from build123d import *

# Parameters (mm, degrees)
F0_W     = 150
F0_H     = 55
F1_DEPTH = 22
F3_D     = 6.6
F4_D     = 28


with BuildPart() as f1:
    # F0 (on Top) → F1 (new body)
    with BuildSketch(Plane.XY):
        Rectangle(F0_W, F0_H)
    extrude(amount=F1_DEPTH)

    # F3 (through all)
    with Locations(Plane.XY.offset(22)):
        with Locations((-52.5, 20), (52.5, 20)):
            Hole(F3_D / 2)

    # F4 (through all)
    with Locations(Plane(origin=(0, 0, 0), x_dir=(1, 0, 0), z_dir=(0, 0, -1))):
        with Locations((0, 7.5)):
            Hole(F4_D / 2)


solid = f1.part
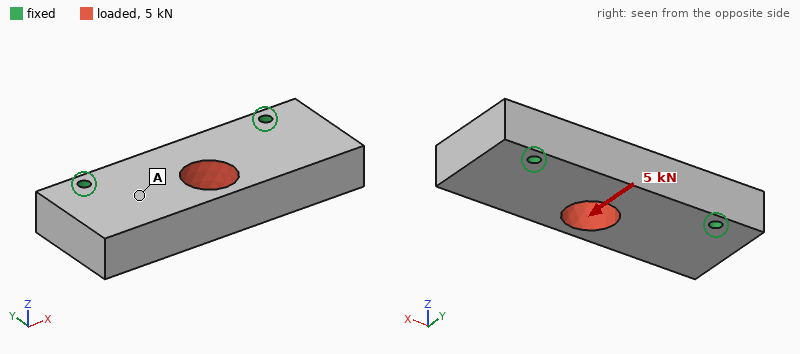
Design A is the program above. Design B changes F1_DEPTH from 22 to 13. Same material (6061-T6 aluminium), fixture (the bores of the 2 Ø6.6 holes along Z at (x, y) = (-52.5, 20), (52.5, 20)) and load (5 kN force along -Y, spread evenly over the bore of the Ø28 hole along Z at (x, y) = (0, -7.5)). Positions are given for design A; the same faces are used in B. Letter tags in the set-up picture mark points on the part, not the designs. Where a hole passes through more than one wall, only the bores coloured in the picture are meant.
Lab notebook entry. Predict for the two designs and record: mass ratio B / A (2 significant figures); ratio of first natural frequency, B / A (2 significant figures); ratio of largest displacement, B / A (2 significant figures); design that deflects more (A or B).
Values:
0.59
0.69
1.7
B
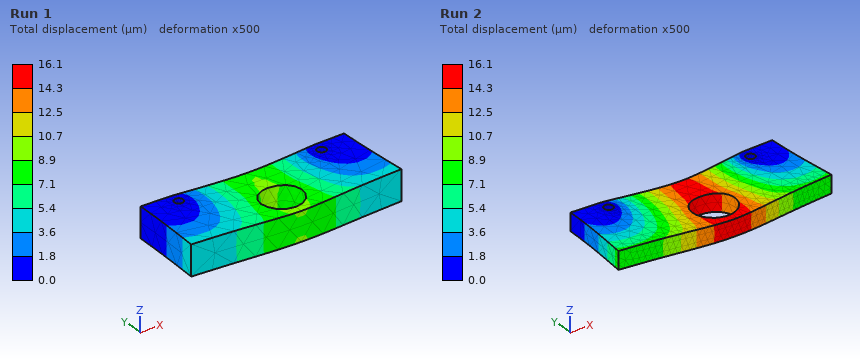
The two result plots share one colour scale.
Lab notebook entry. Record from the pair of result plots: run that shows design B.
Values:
Run 2
